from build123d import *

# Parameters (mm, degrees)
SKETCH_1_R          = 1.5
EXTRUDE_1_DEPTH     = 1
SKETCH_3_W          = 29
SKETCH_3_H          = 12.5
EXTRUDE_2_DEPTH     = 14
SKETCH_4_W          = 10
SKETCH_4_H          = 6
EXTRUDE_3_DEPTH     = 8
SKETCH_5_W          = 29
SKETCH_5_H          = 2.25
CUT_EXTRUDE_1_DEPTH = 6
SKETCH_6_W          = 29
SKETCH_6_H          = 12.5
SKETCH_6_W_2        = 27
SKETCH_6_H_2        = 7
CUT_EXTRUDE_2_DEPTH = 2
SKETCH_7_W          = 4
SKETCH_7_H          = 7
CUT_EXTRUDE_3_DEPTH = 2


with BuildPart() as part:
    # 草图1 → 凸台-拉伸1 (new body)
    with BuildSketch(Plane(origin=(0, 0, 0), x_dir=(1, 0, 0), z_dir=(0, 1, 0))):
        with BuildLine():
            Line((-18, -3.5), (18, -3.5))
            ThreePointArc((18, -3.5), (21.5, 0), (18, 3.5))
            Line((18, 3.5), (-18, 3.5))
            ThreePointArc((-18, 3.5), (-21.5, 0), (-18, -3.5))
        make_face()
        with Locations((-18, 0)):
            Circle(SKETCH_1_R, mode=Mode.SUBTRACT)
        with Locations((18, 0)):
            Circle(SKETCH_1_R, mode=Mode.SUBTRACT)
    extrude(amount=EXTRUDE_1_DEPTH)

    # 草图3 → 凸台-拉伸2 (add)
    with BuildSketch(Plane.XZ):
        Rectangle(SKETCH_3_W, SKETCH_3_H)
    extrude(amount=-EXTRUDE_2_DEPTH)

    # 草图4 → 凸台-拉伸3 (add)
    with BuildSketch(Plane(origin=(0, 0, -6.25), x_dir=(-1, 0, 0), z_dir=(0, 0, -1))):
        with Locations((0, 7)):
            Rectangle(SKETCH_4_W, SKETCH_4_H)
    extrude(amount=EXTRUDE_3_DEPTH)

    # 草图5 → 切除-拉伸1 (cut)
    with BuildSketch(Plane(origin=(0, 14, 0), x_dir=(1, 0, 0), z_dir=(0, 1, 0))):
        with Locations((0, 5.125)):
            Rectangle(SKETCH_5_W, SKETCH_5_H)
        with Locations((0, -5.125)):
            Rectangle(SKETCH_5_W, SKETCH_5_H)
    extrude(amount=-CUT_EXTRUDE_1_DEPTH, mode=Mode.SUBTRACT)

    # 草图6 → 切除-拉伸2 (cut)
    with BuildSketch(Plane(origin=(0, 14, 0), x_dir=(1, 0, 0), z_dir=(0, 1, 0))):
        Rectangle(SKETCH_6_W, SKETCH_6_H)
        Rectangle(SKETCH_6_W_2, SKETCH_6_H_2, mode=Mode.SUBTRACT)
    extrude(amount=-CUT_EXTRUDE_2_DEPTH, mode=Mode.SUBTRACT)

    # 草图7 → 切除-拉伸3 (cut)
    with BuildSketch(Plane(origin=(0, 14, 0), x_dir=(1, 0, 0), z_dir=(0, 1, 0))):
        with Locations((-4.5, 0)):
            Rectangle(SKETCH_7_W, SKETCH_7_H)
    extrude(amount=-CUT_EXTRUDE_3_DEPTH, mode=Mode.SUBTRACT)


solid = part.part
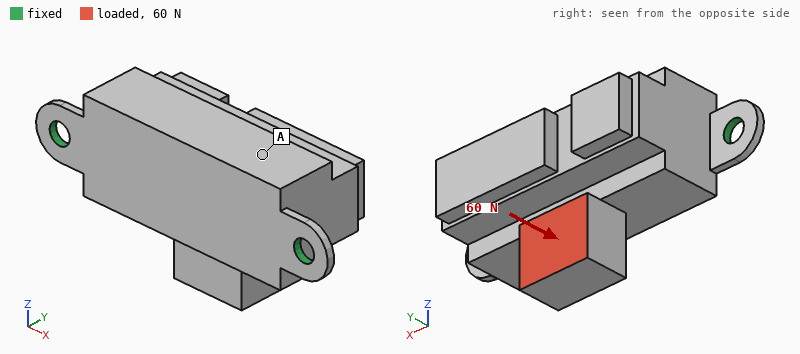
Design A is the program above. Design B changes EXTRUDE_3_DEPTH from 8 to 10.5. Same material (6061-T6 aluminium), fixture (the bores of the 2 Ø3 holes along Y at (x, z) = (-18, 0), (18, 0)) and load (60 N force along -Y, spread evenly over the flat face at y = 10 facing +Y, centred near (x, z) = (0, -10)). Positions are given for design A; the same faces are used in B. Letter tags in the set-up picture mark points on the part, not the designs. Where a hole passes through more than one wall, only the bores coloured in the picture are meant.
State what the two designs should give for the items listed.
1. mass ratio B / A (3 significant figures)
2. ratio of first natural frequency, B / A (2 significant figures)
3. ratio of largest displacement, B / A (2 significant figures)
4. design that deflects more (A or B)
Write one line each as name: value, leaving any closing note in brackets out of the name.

mass ratio B / A: 1.03
ratio of first natural frequency, B / A: 0.94
ratio of largest displacement, B / A: 1.3
design that deflects more: B
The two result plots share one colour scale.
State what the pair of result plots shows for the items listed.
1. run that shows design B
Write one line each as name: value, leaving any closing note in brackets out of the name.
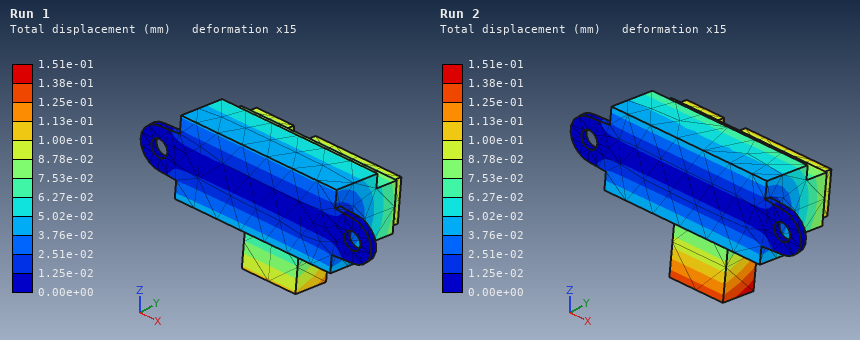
run that shows design B: Run 2
